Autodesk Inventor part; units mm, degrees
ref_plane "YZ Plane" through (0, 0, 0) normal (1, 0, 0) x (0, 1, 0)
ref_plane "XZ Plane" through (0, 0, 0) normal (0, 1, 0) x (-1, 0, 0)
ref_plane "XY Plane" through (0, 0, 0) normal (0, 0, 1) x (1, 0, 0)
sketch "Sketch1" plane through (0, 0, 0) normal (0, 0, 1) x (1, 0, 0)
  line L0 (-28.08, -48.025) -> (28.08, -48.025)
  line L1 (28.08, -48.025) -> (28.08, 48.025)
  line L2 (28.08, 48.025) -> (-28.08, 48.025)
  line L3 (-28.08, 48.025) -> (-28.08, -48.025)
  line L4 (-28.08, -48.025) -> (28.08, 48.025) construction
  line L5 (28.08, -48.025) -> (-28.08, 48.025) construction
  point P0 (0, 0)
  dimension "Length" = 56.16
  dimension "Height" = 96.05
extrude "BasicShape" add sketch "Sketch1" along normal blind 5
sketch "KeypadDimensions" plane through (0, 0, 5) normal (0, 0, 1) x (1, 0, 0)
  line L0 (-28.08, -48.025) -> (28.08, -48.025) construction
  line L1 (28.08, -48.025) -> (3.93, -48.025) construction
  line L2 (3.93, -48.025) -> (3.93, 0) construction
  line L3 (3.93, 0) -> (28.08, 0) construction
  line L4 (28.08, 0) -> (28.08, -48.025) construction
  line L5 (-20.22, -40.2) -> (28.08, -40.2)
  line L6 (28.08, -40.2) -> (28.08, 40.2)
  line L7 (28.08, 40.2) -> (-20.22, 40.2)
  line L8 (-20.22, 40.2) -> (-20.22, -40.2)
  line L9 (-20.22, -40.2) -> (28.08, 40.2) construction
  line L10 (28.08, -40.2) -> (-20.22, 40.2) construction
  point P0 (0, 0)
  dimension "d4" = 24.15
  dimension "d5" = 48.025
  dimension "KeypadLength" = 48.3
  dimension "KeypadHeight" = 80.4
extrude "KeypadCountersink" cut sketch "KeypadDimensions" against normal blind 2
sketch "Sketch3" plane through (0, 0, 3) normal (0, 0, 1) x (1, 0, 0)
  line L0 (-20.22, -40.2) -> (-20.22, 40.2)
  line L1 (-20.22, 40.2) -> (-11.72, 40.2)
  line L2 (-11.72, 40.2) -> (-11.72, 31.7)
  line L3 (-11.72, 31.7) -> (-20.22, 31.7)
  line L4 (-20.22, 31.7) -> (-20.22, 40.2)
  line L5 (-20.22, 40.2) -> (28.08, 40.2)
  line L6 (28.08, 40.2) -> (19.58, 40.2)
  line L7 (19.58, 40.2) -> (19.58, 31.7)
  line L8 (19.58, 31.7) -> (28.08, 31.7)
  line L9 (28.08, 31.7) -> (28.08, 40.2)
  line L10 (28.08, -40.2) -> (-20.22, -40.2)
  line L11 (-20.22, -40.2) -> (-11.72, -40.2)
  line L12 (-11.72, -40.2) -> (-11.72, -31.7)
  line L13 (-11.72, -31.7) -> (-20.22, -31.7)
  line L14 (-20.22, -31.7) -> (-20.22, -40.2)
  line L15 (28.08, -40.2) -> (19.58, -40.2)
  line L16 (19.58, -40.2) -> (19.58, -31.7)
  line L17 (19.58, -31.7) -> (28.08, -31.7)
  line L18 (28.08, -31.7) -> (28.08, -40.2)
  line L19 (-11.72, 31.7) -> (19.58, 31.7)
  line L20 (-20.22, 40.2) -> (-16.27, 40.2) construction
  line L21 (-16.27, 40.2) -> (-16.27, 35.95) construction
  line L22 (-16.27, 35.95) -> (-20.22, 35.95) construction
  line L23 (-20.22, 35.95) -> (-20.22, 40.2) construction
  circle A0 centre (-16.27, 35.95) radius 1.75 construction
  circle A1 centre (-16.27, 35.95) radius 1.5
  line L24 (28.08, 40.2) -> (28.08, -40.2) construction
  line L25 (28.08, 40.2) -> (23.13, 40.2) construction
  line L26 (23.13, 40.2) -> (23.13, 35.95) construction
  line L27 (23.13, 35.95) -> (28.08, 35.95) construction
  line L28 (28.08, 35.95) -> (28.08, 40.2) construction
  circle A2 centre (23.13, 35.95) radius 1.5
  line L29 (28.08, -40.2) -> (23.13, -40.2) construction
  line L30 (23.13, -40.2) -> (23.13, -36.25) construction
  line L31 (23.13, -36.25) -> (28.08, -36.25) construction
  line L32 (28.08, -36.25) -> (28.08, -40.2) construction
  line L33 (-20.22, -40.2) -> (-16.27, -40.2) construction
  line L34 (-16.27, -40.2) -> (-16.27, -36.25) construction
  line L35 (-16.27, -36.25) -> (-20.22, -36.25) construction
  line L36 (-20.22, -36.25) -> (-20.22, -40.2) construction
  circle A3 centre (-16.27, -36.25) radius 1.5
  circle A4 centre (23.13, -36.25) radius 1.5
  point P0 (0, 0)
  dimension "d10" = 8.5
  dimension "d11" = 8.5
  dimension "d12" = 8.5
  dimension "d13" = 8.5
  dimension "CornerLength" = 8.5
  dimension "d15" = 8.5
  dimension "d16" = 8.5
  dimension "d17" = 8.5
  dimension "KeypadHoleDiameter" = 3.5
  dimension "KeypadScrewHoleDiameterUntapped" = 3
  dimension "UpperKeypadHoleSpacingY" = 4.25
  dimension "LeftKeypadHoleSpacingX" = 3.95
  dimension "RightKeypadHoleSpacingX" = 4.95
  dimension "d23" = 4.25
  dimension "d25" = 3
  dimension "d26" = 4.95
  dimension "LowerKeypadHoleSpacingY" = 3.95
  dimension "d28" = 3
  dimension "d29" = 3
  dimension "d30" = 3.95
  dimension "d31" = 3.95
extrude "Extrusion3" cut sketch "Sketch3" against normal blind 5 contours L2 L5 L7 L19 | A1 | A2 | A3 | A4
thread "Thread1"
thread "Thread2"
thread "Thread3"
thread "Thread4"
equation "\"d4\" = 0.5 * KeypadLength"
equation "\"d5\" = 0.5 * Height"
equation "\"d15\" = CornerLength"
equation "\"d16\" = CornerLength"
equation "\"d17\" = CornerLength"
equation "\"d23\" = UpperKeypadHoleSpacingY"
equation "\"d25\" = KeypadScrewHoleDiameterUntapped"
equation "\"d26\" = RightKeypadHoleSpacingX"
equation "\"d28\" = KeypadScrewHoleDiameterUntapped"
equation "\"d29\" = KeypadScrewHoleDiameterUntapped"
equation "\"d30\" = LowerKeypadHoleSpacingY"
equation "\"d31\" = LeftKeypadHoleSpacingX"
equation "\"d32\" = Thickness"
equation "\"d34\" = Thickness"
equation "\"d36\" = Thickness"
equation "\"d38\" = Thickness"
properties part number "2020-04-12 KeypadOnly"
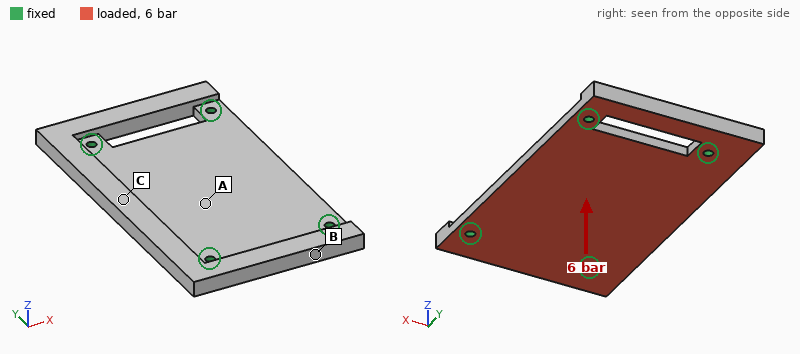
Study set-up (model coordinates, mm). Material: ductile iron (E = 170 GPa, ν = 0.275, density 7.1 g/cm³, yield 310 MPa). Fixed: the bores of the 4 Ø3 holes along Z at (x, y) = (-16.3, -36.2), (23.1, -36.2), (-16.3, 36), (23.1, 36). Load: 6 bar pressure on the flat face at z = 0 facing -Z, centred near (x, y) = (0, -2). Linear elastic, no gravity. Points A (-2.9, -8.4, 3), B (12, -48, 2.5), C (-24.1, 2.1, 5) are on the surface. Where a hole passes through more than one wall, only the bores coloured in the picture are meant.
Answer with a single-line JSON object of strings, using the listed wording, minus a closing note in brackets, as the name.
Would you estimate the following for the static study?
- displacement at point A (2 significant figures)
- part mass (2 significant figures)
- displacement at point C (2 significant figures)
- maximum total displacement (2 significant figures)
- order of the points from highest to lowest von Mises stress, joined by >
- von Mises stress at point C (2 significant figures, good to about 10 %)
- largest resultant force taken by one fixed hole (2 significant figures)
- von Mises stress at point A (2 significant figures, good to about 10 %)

{"displacement at point A": "0.11 mm", "part mass": "130 g", "displacement at point C": "0.082 mm", "maximum total displacement": "0.15 mm", "order of the points from highest to lowest von Mises stress, joined by >": "C > A > B", "von Mises stress at point C": "100 MPa", "largest resultant force taken by one fixed hole": "980 N", "von Mises stress at point A": "57 MPa"}
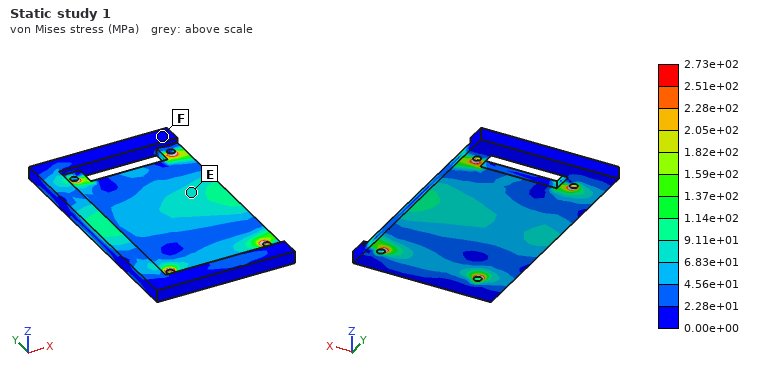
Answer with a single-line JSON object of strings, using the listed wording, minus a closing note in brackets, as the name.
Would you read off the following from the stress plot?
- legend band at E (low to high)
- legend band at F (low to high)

{"legend band at E": "6.83e+01 to 9.11e+01 MPa", "legend band at F": "0.00e+00 to 2.28e+01 MPa"}
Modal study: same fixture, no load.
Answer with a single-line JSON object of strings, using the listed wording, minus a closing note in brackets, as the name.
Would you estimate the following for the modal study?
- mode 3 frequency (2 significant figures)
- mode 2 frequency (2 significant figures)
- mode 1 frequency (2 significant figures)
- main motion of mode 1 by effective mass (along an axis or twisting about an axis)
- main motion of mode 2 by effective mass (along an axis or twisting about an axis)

{"mode 3 frequency": "6300 Hz", "mode 2 frequency": "3800 Hz", "mode 1 frequency": "2600 Hz", "main motion of mode 1 by effective mass": "along Z", "main motion of mode 2 by effective mass": "twisting about Y"}
